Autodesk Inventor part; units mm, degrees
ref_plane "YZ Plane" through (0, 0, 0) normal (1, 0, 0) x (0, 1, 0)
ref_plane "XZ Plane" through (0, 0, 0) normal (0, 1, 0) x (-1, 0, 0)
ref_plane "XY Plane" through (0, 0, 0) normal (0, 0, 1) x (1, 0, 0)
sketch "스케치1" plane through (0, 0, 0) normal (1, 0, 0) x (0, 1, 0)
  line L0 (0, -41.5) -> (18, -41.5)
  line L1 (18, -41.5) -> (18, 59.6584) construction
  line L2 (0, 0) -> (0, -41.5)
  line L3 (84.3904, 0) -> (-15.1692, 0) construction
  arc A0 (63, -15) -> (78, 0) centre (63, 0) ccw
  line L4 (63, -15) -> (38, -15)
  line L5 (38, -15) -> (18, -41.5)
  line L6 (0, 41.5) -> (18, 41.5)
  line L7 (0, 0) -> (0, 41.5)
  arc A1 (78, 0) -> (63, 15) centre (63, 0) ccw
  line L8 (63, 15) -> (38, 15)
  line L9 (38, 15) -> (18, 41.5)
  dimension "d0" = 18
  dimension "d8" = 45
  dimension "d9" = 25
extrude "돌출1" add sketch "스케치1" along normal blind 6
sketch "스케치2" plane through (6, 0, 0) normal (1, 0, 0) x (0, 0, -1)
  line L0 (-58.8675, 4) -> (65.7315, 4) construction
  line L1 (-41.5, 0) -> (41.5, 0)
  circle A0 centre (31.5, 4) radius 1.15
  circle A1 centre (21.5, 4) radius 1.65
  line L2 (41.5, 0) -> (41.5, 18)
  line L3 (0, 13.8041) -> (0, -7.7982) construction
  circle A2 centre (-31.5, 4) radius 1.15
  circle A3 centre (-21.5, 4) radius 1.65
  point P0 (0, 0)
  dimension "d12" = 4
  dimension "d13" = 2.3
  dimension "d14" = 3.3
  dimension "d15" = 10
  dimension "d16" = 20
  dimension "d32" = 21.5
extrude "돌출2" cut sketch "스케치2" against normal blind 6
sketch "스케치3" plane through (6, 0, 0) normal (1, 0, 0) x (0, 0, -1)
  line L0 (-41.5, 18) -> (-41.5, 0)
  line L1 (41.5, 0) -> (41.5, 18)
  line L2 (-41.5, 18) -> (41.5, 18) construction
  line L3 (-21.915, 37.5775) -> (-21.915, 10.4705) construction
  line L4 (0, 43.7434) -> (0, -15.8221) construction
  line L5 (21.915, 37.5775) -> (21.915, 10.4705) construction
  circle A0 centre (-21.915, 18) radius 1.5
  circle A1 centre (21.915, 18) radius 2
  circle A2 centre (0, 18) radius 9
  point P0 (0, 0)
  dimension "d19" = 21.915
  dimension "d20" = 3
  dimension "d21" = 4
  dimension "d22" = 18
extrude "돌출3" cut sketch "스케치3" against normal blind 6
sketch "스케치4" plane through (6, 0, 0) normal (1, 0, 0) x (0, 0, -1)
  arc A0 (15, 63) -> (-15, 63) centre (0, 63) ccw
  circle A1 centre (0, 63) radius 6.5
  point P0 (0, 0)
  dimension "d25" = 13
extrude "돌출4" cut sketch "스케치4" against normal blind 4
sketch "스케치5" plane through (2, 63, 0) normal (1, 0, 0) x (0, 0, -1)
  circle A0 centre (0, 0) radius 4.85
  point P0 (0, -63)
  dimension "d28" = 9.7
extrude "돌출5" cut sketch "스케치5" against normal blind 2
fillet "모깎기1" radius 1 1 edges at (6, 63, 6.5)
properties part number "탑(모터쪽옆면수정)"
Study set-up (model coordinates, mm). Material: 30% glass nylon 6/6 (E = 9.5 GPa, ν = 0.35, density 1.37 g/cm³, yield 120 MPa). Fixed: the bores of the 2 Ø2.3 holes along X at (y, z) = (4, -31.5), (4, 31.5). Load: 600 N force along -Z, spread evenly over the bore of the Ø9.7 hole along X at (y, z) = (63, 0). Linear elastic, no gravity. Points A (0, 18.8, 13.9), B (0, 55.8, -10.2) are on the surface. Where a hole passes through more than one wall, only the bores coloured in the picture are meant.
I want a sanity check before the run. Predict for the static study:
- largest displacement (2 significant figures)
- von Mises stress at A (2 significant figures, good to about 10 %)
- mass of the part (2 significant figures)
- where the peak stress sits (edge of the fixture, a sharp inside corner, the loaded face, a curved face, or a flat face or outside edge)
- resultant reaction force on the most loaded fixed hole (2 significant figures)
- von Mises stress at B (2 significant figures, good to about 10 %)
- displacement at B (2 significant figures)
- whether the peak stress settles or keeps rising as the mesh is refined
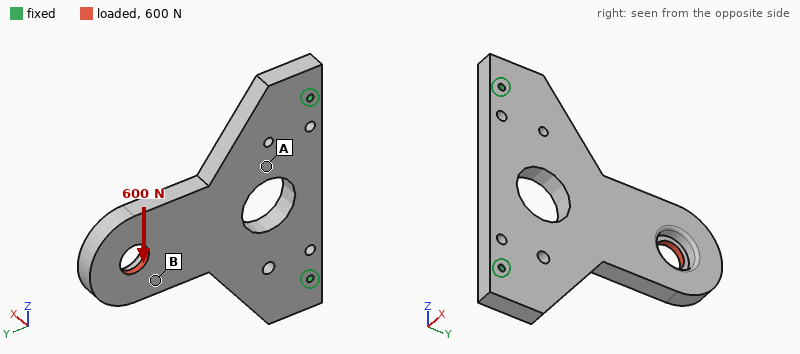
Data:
0.23 mm
4.7 MPa
27 g
edge of the fixture
630 N
11 MPa
0.14 mm
keeps rising
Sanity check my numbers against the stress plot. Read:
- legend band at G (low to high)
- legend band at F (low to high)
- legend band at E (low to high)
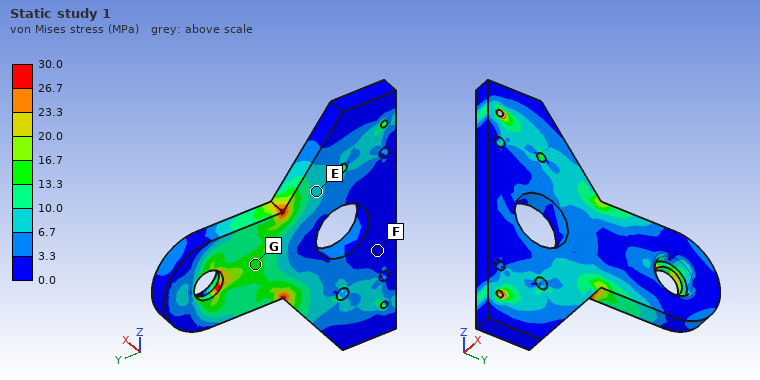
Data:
13.3 to 16.7 MPa
0.0 to 3.3 MPa
6.7 to 10.0 MPa
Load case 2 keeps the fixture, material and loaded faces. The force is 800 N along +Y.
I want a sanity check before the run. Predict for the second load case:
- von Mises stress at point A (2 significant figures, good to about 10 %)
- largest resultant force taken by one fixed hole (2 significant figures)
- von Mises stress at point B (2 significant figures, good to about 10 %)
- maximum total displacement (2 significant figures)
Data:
9.5 MPa
450 N
13 MPa
0.81 mm
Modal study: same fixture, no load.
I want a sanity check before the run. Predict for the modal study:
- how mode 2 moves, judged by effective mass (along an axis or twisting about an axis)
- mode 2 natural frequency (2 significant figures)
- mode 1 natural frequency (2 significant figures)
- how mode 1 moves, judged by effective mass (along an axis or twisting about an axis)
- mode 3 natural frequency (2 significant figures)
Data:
along X
2300 Hz
520 Hz
along X
2600 Hz
